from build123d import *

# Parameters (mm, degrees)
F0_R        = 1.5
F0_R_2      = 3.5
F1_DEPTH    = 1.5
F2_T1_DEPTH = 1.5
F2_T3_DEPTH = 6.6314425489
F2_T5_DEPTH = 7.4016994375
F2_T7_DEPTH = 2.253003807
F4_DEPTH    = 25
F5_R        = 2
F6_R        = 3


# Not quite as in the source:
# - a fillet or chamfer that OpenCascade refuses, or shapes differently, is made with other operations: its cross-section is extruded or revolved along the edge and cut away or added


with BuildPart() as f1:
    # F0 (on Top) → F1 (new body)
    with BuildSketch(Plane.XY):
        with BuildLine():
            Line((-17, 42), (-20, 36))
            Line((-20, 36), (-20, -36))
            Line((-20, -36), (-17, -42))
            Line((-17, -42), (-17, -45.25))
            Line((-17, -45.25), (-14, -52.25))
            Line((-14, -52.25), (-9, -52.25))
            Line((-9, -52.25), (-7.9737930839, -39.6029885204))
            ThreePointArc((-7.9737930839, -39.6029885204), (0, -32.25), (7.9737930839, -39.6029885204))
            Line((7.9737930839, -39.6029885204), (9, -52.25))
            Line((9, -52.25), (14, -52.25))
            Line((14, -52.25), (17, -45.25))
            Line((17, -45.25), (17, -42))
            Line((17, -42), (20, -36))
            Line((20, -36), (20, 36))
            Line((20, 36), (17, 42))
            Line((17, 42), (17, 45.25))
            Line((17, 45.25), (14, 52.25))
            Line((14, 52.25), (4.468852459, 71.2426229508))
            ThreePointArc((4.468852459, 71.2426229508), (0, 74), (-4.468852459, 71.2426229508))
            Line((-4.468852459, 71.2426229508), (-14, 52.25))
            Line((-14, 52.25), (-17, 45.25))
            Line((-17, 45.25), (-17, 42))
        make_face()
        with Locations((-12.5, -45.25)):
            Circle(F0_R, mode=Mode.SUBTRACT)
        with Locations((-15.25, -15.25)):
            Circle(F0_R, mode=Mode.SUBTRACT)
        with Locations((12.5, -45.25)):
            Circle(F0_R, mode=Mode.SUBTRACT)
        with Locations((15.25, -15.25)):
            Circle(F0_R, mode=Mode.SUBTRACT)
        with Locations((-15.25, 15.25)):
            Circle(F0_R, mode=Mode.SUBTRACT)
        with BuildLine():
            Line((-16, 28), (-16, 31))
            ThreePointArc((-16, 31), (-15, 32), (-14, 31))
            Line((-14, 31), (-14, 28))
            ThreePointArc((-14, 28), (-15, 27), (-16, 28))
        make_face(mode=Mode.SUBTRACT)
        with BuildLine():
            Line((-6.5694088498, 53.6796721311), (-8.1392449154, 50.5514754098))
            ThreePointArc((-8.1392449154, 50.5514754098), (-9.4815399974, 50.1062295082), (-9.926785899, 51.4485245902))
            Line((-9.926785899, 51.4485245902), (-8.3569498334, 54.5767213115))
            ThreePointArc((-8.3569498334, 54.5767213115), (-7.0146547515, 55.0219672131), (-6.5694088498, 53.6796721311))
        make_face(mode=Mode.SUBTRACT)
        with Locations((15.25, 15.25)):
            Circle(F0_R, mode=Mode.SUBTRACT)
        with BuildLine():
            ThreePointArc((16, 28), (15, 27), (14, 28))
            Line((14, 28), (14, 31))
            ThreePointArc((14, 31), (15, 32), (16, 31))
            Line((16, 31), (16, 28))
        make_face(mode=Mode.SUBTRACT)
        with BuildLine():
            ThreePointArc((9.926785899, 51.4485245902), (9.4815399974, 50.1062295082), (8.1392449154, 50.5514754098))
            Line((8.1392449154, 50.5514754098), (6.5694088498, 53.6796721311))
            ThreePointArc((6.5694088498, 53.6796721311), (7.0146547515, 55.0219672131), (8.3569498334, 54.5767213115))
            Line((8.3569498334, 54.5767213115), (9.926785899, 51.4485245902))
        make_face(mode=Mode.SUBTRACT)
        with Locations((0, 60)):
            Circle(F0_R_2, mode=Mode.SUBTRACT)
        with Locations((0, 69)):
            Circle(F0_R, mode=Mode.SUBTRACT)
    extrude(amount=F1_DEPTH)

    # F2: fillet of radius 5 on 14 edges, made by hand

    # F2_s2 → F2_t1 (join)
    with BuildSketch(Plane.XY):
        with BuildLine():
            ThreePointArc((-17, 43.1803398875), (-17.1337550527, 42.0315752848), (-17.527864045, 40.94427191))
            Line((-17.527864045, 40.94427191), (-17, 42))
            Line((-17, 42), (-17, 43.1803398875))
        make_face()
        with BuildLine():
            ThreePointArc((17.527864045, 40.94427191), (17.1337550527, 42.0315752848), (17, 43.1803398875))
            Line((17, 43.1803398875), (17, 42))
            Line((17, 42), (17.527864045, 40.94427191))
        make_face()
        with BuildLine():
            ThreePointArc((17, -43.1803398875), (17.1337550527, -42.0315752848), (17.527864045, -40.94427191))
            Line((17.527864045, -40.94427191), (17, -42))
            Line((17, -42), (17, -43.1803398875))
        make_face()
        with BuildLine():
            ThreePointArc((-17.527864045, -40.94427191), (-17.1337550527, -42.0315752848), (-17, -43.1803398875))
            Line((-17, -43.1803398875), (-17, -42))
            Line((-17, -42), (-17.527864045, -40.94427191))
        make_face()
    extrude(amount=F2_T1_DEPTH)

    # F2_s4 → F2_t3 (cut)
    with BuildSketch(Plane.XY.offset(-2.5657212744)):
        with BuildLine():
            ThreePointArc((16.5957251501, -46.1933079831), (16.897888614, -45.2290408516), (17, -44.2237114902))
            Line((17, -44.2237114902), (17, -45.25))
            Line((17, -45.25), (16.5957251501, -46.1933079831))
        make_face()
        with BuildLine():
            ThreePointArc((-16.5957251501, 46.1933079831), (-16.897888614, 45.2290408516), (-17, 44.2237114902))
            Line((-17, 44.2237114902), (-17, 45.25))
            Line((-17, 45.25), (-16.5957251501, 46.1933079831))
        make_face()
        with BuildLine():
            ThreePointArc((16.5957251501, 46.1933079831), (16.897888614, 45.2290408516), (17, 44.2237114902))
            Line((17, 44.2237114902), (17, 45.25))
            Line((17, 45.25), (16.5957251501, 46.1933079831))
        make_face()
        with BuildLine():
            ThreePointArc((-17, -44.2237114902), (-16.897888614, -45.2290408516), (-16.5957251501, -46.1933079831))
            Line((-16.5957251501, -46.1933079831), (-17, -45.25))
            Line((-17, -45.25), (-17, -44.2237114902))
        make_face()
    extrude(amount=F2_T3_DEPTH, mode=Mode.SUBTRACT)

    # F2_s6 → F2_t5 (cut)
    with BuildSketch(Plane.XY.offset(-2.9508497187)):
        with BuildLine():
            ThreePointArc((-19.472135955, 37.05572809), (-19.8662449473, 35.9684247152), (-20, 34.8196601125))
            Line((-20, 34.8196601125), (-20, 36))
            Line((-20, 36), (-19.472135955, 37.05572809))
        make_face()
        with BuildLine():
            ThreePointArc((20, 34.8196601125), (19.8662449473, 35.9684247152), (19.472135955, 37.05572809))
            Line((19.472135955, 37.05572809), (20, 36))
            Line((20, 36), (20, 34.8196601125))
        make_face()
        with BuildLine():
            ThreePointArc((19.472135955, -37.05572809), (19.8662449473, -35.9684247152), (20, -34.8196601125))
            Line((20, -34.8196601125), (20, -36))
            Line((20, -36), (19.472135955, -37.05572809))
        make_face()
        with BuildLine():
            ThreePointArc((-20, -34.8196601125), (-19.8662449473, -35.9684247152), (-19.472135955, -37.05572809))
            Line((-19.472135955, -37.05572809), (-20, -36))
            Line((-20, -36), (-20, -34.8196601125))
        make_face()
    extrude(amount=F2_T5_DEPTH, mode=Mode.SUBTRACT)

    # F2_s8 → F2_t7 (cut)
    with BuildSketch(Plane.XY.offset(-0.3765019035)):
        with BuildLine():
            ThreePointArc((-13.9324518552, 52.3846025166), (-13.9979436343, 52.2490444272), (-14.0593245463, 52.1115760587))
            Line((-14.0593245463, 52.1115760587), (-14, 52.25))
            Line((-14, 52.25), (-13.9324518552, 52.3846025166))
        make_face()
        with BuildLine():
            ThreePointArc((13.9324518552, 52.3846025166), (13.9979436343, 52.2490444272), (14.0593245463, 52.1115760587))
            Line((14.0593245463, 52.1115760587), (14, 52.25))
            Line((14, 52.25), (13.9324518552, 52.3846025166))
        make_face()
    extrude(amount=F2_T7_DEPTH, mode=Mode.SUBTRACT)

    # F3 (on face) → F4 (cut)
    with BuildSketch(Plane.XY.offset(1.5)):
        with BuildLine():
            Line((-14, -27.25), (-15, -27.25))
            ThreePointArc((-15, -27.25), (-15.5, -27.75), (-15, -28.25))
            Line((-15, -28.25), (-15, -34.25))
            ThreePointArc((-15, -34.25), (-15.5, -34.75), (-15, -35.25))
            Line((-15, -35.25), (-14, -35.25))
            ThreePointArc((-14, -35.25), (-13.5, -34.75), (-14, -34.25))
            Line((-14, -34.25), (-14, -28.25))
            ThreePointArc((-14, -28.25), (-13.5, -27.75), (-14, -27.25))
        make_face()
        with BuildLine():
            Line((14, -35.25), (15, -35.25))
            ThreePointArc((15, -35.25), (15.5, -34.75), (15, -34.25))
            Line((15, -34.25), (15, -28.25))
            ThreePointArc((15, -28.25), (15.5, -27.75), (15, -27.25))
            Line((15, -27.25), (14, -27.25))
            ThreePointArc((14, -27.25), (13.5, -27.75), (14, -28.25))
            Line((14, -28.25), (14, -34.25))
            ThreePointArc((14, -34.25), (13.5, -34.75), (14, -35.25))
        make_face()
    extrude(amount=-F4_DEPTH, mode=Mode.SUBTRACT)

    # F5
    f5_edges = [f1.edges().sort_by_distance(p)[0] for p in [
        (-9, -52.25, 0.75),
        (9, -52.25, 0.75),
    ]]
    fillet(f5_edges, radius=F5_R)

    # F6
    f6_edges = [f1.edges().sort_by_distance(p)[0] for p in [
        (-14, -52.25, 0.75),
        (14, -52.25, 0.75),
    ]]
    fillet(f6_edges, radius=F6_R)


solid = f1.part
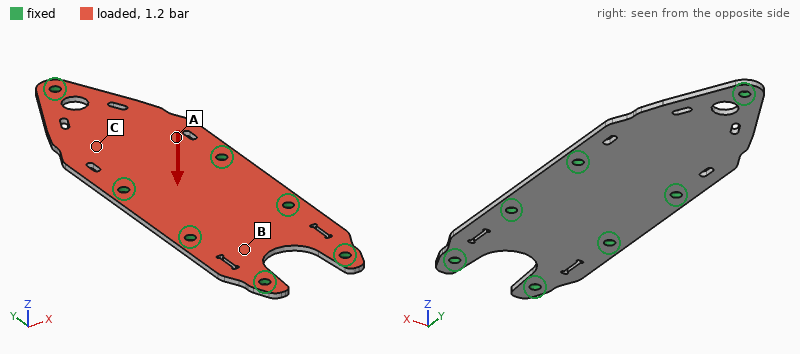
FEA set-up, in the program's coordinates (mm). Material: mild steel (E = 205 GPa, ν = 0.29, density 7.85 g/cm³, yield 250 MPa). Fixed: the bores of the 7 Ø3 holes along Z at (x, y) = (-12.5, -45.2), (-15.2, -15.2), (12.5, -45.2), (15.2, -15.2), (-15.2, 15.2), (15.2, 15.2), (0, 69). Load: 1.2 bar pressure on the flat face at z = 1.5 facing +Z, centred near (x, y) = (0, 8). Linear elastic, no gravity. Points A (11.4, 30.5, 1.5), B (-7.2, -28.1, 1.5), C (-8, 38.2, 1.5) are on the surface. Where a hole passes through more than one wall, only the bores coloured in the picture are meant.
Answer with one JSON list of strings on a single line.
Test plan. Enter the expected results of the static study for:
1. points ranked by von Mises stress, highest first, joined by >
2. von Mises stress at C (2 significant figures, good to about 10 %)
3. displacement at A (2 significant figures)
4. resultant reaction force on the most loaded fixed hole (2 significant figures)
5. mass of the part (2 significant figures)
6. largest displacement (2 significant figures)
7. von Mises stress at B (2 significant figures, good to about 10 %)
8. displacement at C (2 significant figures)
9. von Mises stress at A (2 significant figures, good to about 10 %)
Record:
["C > A > B", "33 MPa", "36 µm", "100 N", "46 g", "62 µm", "9.2 MPa", "52 µm", "18 MPa"]
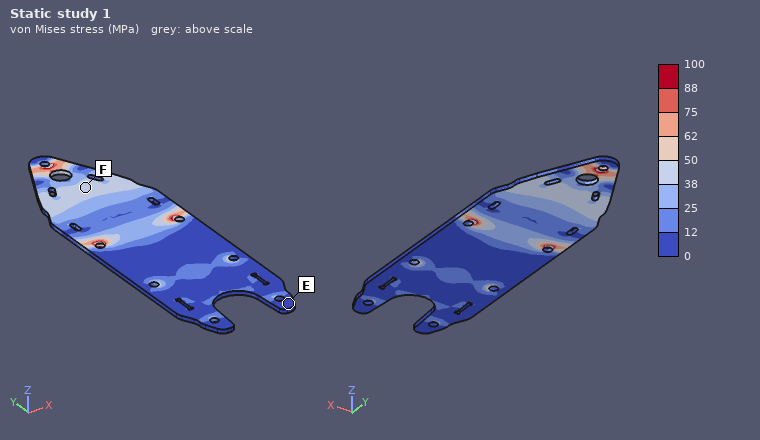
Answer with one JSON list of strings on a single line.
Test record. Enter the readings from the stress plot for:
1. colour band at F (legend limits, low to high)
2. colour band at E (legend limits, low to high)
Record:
["38 to 50 MPa", "0 to 12 MPa"]
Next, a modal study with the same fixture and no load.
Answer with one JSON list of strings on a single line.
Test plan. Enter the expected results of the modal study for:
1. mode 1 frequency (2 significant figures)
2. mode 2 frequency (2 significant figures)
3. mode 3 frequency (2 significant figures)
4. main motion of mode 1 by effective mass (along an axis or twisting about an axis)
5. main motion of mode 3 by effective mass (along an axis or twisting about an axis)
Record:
["2400 Hz", "3200 Hz", "6400 Hz", "along Z", "along Z"]
